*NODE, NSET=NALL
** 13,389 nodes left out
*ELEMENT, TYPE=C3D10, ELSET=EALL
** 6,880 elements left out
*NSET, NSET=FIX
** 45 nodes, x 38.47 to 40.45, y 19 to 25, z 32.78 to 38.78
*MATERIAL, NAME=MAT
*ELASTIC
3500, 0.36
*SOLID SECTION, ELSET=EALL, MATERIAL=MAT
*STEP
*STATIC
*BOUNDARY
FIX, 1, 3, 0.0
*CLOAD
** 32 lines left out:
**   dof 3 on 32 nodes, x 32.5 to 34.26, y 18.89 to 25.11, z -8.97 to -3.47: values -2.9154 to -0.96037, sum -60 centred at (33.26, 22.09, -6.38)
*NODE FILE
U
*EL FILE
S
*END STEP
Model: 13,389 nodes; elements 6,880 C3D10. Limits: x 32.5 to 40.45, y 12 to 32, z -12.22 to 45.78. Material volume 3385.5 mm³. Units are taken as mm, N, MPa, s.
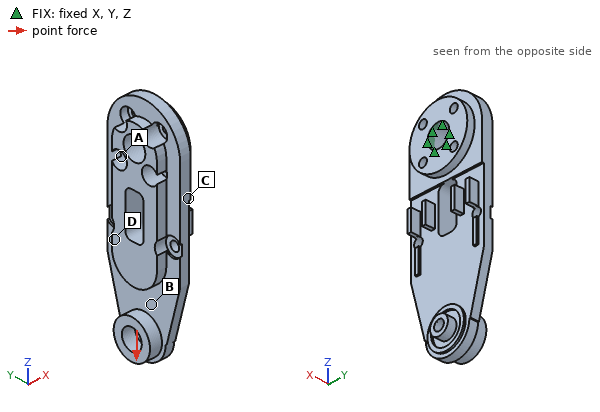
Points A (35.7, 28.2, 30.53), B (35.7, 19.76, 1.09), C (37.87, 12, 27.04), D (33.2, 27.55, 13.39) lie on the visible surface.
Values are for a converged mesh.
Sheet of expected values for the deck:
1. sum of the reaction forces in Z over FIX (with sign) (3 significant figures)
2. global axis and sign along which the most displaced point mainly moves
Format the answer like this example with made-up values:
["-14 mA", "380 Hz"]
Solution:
["60.0 N", "+X"]
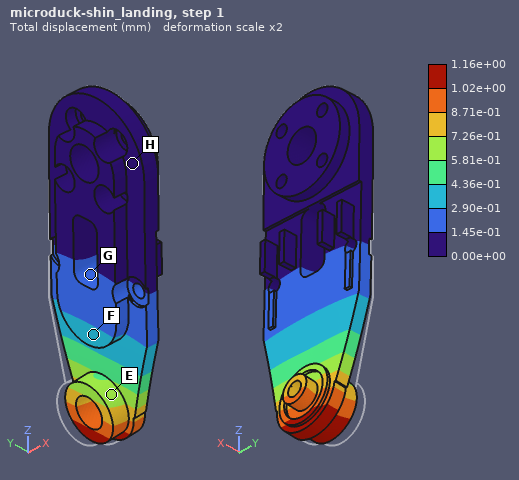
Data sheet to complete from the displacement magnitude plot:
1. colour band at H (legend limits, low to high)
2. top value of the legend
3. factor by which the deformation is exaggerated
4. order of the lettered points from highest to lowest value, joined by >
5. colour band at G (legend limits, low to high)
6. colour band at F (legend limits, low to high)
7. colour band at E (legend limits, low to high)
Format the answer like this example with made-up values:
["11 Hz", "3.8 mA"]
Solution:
["0.00e+00 to 1.45e-01 mm", "1.16e+00 mm", "2", "E > F > G > H", "1.45e-01 to 2.90e-01 mm", "2.90e-01 to 4.36e-01 mm", "5.81e-01 to 7.26e-01 mm"]
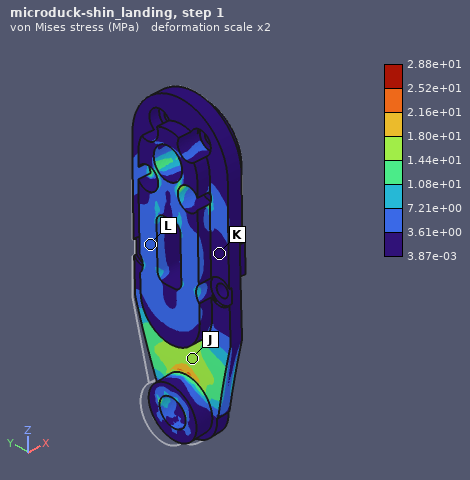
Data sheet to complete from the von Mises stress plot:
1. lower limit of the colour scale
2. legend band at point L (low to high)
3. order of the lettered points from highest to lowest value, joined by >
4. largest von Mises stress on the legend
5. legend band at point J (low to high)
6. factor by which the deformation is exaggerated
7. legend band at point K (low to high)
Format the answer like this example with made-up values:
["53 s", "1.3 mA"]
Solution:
["3.87e-03 MPa", "3.61e+00 to 7.21e+00 MPa", "J > L > K", "2.88e+01 MPa", "1.44e+01 to 1.80e+01 MPa", "2", "3.87e-03 to 3.61e+00 MPa"]
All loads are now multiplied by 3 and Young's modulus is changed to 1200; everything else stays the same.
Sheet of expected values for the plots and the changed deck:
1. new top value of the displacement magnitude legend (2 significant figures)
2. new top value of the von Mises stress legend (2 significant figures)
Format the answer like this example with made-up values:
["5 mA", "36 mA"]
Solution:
["10 mm", "86 MPa"]
